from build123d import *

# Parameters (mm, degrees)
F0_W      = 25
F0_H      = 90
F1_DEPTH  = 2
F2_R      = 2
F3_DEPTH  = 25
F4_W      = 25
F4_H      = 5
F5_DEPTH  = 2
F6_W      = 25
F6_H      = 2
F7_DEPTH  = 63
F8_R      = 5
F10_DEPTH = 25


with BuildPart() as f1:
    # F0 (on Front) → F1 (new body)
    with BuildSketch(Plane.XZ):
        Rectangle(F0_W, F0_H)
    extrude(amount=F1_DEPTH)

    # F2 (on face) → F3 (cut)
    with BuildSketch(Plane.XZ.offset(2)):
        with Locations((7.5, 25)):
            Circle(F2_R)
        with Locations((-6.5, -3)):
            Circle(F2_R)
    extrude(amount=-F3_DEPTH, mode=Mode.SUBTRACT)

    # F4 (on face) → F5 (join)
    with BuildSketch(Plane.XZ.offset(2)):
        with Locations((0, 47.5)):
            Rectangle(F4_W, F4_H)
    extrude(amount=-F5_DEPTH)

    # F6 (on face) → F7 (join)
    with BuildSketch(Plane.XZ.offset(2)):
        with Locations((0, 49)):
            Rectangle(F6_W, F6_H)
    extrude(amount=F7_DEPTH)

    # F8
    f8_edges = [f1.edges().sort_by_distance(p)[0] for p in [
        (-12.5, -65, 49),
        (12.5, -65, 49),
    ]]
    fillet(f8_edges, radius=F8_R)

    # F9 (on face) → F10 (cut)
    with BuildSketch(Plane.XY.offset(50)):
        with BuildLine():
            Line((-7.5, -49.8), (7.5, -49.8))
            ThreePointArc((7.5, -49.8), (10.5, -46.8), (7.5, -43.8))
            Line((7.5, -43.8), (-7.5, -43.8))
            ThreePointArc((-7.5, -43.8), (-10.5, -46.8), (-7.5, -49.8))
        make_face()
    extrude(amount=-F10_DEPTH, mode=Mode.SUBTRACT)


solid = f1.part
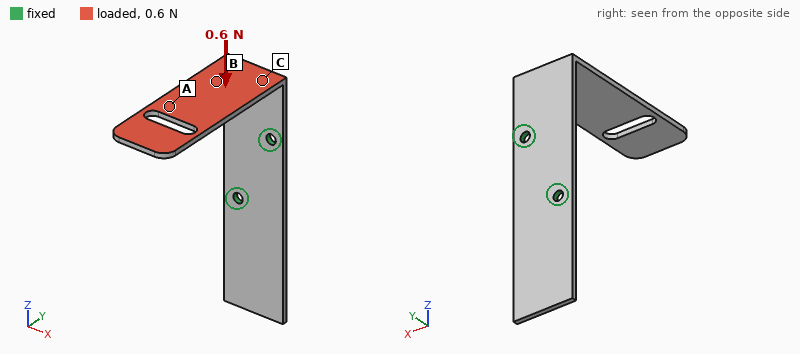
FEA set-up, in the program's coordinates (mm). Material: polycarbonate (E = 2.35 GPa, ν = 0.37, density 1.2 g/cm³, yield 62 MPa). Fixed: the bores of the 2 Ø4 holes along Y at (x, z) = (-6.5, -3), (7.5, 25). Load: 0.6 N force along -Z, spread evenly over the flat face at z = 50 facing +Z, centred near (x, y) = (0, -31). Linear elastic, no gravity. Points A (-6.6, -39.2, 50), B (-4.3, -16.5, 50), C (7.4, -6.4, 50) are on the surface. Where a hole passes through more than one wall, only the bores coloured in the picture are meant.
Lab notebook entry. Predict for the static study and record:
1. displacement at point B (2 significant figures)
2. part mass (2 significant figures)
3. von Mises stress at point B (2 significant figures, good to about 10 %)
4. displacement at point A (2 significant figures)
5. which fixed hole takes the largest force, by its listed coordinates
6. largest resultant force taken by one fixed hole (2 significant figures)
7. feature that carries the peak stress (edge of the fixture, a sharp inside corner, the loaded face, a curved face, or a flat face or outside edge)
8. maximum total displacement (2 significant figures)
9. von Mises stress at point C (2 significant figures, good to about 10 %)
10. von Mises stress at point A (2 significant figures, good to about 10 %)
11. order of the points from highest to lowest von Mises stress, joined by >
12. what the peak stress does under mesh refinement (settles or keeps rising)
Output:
0.26 mm
9.1 g
0.56 MPa
0.62 mm
(7.5, 25)
0.48 N
edge of the fixture
1.2 mm
0.83 MPa
0.20 MPa
C > B > A
keeps rising
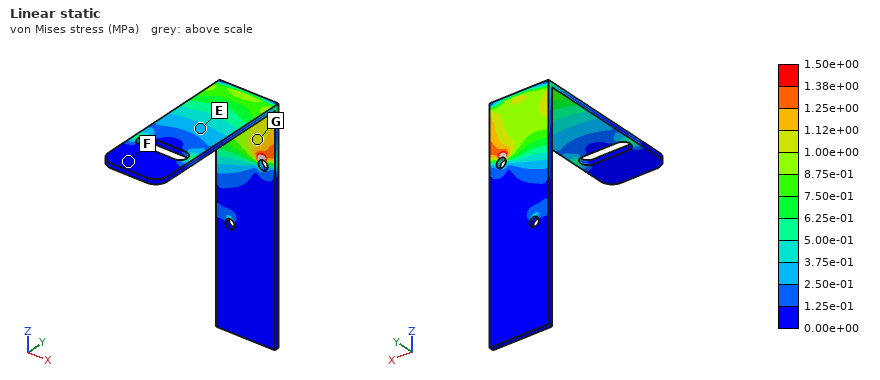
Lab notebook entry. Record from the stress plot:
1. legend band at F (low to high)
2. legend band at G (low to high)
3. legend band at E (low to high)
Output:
0.00e+00 to 1.25e-01 MPa
1.00e+00 to 1.12e+00 MPa
2.50e-01 to 3.75e-01 MPa
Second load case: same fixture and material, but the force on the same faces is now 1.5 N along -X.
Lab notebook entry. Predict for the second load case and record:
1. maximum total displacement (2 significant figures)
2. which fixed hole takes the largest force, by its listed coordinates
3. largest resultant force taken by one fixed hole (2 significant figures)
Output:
1.2 mm
(7.5, 25)
2.4 N
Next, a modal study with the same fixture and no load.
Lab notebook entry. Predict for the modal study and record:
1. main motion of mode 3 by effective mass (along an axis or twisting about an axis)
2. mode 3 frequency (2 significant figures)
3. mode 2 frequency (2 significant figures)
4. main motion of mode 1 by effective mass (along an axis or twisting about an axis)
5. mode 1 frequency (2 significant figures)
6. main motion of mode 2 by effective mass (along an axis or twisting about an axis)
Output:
along Y
250 Hz
110 Hz
along Z
74 Hz
along X
